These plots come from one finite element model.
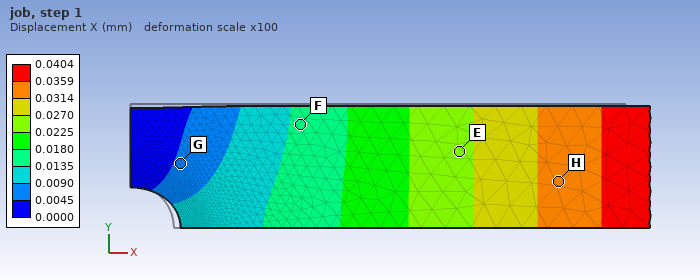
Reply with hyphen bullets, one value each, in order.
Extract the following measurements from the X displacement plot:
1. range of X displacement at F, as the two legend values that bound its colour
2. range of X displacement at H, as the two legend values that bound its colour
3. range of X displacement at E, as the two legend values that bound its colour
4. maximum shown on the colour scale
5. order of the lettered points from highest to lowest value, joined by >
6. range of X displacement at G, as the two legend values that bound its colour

- 0.0135 to 0.0180 mm
- 0.0314 to 0.0359 mm
- 0.0225 to 0.0270 mm
- 0.0404 mm
- H > E > F > G
- 0.0045 to 0.0090 mm
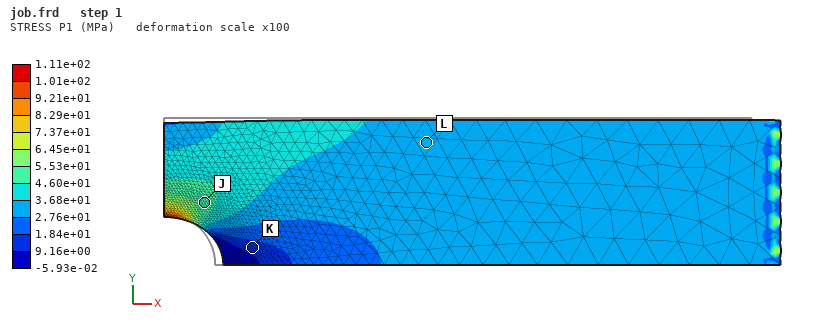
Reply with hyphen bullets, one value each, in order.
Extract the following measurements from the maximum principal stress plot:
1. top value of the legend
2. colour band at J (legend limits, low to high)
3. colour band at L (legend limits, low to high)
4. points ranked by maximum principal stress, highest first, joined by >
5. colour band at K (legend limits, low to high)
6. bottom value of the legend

- 1.11e+02 MPa
- 4.60e+01 to 5.53e+01 MPa
- 2.76e+01 to 3.68e+01 MPa
- J > L > K
- 9.16e+00 to 1.84e+01 MPa
- -5.93e-02 MPa
